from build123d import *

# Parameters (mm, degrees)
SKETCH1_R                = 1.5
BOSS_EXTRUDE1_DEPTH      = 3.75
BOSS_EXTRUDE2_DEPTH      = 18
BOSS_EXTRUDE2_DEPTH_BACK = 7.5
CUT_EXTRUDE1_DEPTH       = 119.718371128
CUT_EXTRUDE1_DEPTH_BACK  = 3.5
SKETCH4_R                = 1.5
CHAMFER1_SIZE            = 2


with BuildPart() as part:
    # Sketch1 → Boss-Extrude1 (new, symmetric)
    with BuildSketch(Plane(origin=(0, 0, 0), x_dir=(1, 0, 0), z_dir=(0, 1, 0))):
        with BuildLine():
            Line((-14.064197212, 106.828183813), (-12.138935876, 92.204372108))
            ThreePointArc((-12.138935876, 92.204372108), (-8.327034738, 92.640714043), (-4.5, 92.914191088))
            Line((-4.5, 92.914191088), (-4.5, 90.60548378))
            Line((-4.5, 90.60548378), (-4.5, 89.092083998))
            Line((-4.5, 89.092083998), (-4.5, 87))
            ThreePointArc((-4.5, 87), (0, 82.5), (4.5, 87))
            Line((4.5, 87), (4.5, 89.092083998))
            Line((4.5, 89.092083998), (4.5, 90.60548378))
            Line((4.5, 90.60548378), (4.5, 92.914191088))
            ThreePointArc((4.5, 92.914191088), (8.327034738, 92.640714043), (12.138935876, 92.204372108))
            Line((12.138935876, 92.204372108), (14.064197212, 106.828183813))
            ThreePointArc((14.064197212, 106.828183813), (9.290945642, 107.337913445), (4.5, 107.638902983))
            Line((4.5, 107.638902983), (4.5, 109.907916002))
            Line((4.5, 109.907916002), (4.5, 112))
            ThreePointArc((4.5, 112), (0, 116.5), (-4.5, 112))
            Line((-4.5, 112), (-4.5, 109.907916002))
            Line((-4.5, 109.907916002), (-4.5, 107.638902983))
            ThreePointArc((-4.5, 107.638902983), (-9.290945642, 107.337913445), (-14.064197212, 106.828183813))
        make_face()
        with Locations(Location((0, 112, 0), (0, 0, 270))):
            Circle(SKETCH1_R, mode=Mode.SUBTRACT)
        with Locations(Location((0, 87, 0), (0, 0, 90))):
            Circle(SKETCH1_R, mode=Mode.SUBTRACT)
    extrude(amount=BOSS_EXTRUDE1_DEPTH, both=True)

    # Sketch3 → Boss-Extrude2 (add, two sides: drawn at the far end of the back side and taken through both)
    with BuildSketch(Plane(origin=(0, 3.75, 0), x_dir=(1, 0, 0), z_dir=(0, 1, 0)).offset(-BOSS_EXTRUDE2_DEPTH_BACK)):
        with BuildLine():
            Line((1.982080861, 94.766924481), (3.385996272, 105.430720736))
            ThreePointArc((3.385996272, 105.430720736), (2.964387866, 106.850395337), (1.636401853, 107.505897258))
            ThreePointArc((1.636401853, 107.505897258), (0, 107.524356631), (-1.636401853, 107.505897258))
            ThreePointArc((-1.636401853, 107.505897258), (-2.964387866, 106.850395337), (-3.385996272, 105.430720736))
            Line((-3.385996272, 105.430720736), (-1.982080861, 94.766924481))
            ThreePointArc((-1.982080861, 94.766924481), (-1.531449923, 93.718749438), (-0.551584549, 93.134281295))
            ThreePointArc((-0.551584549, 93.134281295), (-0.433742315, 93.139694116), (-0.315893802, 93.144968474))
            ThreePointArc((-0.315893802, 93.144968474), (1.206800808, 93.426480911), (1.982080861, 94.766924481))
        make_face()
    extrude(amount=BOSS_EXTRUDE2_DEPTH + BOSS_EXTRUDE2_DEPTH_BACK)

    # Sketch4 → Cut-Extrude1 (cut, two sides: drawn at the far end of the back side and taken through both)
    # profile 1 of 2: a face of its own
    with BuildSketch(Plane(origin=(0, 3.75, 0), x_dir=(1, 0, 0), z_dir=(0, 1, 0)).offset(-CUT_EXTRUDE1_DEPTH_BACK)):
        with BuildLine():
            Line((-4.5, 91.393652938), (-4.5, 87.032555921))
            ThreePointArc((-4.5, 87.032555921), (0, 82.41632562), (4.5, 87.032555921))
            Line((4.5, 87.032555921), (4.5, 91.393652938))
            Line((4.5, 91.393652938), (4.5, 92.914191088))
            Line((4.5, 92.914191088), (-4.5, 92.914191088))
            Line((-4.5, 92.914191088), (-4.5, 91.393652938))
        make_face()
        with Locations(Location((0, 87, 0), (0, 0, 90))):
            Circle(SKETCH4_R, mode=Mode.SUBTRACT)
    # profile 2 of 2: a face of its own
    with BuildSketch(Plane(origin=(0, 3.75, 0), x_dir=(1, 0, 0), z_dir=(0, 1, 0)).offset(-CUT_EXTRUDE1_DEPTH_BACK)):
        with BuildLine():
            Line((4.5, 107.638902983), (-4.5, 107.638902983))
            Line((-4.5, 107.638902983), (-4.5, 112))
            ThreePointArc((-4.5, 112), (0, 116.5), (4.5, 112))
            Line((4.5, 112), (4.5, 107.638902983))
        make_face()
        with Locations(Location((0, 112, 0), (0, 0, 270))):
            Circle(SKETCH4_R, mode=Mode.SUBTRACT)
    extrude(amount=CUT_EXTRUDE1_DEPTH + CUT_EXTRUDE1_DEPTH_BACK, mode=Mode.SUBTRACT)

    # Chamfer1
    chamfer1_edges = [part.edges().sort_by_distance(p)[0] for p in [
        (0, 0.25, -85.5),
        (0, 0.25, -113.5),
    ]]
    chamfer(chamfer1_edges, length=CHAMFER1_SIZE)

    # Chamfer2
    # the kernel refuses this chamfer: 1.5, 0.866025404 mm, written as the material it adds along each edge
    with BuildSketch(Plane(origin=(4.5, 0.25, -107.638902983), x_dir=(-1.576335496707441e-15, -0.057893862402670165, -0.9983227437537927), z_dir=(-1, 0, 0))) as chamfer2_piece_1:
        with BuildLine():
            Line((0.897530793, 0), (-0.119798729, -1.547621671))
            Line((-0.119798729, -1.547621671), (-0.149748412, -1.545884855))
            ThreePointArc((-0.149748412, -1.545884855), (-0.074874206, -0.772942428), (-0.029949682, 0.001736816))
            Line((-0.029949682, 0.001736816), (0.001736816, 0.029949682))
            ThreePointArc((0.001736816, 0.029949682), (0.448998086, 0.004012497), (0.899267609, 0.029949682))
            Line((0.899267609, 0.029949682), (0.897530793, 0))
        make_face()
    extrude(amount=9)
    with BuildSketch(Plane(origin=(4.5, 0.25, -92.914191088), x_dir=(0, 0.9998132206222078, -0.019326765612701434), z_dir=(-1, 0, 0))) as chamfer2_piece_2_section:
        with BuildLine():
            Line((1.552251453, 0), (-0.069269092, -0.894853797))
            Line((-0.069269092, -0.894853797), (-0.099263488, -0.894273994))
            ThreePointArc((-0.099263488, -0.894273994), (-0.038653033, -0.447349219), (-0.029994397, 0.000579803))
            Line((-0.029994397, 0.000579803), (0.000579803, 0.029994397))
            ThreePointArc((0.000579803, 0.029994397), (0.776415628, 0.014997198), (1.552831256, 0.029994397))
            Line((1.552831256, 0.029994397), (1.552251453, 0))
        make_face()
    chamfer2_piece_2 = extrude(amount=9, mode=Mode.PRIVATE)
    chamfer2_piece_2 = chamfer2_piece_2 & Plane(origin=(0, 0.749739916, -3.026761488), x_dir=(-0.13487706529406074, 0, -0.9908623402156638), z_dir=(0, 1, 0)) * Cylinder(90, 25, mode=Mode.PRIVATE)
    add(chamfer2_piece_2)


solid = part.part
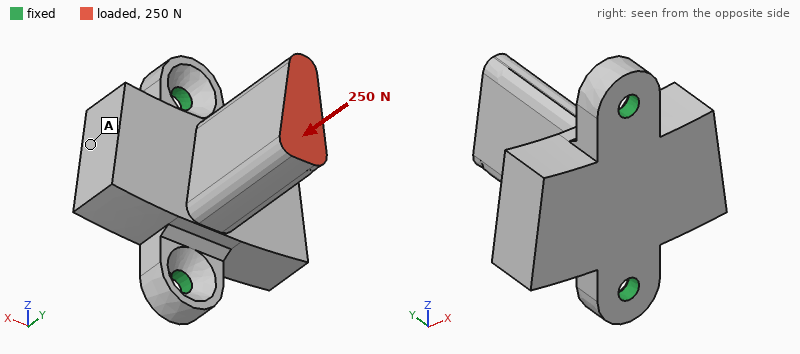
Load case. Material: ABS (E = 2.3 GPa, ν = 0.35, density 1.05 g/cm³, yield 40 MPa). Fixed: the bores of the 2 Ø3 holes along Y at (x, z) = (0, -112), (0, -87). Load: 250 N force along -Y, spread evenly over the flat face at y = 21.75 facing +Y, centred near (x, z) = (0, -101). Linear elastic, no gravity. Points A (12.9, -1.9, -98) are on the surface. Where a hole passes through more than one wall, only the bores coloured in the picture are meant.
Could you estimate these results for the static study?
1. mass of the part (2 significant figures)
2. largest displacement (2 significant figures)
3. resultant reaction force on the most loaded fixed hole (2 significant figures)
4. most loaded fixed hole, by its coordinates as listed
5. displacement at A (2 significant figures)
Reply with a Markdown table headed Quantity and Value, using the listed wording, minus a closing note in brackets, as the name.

| Quantity | Value |
|---|---|
| mass of the part | 5.0 g |
| largest displacement | 94 µm |
| resultant reaction force on the most loaded fixed hole | 170 N |
| most loaded fixed hole, by its coordinates as listed | (0, -112) |
| displacement at A | 68 µm |
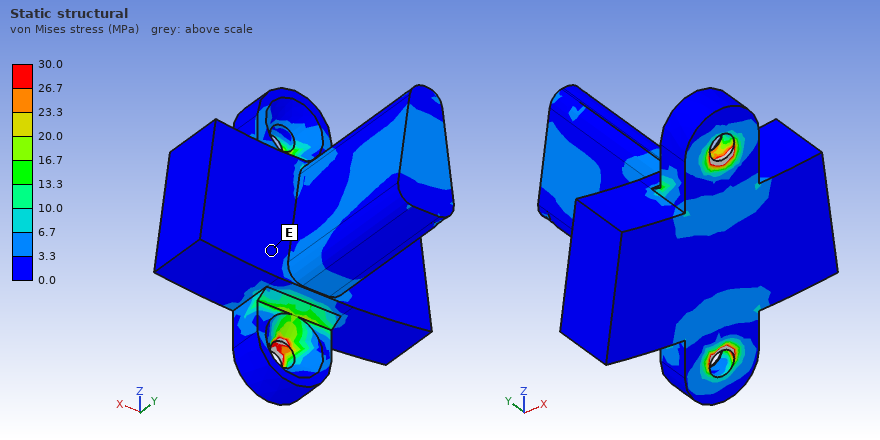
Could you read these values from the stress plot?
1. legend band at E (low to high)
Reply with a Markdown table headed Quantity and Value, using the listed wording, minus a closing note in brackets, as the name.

| Quantity | Value |
|---|---|
| legend band at E | 0.0 to 3.3 MPa |
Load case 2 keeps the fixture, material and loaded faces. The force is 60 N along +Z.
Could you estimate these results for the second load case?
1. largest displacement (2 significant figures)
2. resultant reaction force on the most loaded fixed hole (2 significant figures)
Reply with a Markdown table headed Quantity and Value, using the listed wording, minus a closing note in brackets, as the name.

| Quantity | Value |
|---|---|
| largest displacement | 0.17 mm |
| resultant reaction force on the most loaded fixed hole | 77 N |
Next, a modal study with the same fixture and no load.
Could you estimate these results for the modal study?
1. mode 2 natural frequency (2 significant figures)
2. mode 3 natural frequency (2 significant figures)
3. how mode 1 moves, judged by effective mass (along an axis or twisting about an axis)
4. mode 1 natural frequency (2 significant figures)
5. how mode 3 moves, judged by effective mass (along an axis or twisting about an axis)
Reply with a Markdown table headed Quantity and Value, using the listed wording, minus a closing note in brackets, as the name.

| Quantity | Value |
|---|---|
| mode 2 natural frequency | 4000 Hz |
| mode 3 natural frequency | 4600 Hz |
| how mode 1 moves, judged by effective mass | along X |
| mode 1 natural frequency | 1100 Hz |
| how mode 3 moves, judged by effective mass | along Y |
